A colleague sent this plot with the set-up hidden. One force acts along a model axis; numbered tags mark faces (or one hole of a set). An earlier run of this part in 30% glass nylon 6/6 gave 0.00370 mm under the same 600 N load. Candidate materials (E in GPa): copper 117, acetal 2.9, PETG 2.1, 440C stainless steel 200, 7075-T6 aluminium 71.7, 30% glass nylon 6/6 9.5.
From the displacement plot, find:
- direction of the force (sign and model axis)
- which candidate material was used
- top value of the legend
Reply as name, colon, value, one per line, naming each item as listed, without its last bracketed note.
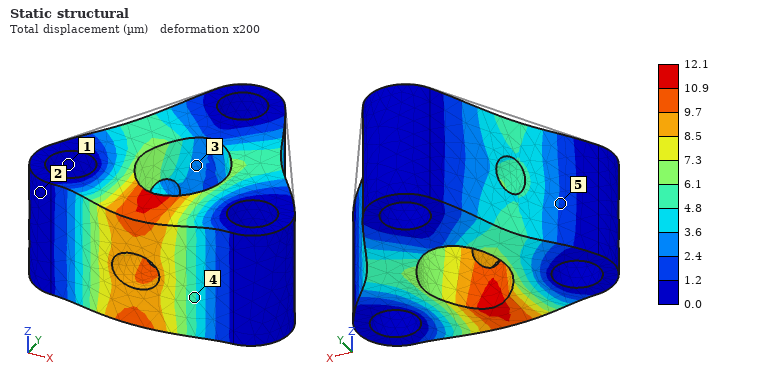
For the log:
direction of the force: -Y
which candidate material was used: acetal
top value of the legend: 12.1 µm
